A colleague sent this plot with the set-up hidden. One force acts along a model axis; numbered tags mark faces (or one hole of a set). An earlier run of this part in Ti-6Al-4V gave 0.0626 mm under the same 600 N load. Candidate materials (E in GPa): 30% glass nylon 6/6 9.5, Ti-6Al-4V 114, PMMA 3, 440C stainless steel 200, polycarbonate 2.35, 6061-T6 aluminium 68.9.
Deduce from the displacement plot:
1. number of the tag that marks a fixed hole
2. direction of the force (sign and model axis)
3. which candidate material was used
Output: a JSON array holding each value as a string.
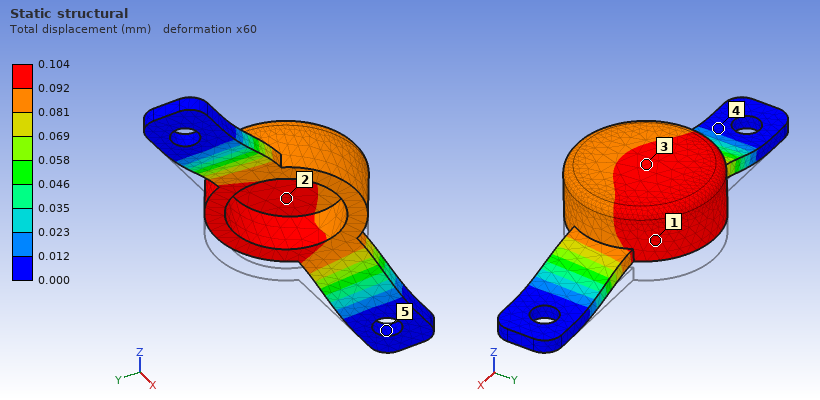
["5", "+Z", "6061-T6 aluminium"]
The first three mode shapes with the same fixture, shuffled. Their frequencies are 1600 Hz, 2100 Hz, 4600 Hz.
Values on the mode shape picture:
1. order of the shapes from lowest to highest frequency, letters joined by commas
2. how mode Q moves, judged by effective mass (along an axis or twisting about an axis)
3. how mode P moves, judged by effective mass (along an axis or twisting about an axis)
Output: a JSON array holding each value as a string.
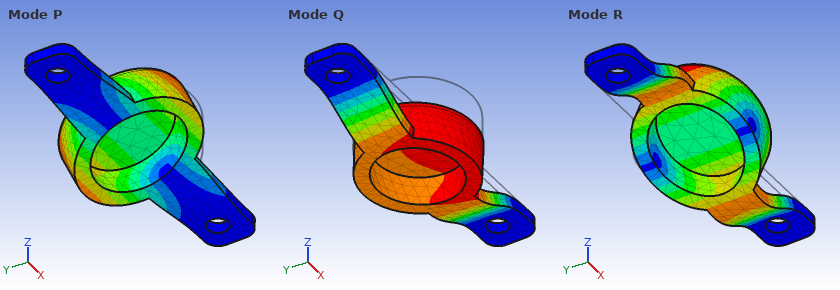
["P, Q, R", "along Z", "along Y"]
